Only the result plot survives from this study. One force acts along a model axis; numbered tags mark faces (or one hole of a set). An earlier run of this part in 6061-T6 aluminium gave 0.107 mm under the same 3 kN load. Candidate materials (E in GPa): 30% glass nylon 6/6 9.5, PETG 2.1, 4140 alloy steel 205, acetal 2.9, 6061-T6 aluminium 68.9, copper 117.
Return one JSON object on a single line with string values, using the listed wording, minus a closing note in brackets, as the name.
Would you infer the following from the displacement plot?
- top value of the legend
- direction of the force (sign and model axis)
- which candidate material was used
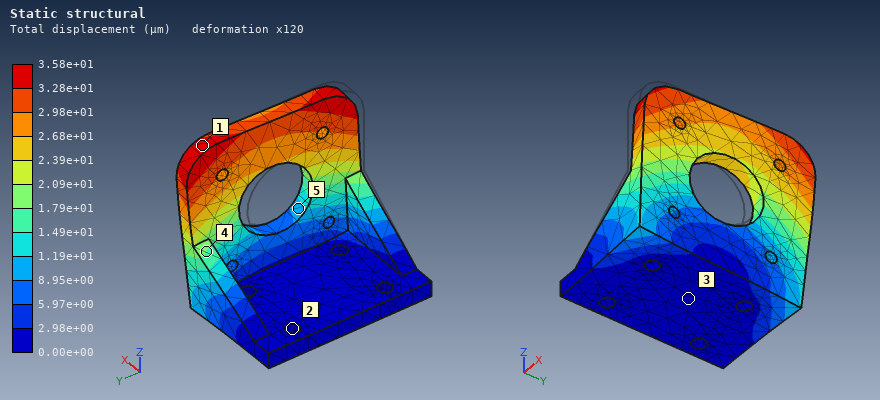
{"top value of the legend": "3.58e+01 µm", "direction of the force": "+Y", "which candidate material was used": "4140 alloy steel"}
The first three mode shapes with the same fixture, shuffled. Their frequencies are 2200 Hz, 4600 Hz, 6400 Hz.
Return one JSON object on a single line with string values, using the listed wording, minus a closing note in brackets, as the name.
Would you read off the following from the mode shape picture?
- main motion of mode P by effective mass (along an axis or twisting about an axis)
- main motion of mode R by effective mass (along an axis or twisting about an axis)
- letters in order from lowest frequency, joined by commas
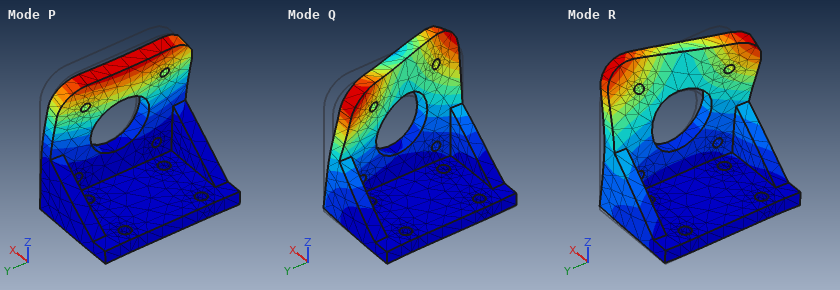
{"main motion of mode P by effective mass": "along X", "main motion of mode R by effective mass": "along Y", "letters in order from lowest frequency, joined by commas": "P, Q, R"}
